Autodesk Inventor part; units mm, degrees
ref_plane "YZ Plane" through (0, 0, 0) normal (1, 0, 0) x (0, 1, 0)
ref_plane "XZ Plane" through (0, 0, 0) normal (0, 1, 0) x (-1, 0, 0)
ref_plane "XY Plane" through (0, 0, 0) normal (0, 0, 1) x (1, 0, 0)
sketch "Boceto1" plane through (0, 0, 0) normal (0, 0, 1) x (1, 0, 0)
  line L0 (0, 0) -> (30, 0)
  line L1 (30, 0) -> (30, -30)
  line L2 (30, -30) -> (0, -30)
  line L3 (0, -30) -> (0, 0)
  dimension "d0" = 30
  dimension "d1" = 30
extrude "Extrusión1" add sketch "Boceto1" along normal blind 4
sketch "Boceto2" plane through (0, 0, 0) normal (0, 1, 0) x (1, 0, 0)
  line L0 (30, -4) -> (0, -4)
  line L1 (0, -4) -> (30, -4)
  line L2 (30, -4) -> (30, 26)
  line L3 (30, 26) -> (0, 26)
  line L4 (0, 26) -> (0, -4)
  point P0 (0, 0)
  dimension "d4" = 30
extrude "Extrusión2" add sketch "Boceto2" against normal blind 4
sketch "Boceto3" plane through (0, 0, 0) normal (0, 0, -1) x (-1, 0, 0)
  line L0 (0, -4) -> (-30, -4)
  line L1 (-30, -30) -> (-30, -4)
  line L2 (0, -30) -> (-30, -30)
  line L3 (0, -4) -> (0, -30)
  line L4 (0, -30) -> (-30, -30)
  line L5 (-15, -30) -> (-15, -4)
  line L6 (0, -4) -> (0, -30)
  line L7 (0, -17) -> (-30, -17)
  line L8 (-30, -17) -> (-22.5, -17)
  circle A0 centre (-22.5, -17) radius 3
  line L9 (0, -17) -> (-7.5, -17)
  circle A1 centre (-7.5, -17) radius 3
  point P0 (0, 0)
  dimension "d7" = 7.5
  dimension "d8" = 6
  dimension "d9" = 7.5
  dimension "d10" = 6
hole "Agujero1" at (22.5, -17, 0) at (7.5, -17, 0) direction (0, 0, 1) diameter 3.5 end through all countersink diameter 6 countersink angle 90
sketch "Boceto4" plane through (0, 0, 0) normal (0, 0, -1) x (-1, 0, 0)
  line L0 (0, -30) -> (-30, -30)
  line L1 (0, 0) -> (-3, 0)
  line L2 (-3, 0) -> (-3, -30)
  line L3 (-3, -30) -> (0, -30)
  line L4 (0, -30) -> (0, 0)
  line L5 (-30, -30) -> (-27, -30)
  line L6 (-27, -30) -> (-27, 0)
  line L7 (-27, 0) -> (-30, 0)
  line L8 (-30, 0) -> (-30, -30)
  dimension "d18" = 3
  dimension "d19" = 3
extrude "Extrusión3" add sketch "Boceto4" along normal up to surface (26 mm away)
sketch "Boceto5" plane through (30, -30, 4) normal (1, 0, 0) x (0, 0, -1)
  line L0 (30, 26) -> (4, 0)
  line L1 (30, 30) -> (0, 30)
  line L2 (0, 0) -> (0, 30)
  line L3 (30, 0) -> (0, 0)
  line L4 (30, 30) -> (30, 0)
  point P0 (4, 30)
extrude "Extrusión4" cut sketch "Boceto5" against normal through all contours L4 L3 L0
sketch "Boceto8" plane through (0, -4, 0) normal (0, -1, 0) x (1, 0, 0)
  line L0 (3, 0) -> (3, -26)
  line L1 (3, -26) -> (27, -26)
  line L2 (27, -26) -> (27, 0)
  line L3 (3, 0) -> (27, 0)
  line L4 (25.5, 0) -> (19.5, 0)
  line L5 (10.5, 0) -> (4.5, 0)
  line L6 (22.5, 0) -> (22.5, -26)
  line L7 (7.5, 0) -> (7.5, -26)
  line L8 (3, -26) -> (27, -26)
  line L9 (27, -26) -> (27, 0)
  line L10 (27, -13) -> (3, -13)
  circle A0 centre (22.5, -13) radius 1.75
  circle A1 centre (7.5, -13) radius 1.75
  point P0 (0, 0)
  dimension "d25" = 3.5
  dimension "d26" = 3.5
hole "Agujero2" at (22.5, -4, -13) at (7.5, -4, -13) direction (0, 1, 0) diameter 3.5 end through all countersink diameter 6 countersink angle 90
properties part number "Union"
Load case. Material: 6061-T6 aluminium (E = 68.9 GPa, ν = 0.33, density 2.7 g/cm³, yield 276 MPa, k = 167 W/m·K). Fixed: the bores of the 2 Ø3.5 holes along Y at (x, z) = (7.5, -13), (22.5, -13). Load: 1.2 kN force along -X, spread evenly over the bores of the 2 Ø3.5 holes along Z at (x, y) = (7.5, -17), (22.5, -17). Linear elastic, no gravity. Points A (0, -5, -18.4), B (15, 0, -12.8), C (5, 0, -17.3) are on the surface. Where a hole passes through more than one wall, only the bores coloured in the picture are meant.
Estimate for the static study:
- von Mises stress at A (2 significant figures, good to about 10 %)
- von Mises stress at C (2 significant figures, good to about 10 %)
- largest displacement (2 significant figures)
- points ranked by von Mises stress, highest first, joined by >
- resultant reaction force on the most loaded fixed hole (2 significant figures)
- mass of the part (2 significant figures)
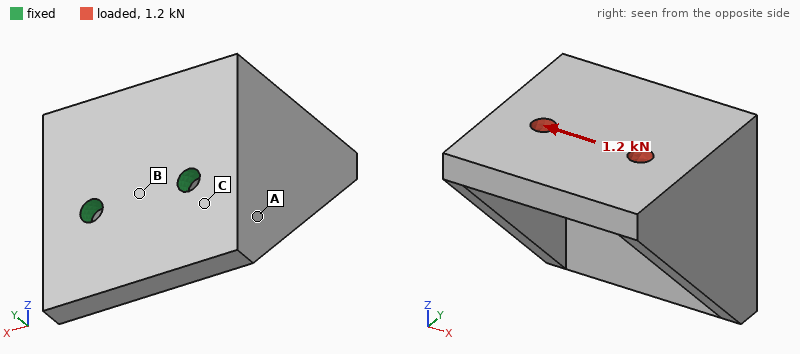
41 MPa
63 MPa
0.15 mm
C > A > B
1.5 kN
23 g
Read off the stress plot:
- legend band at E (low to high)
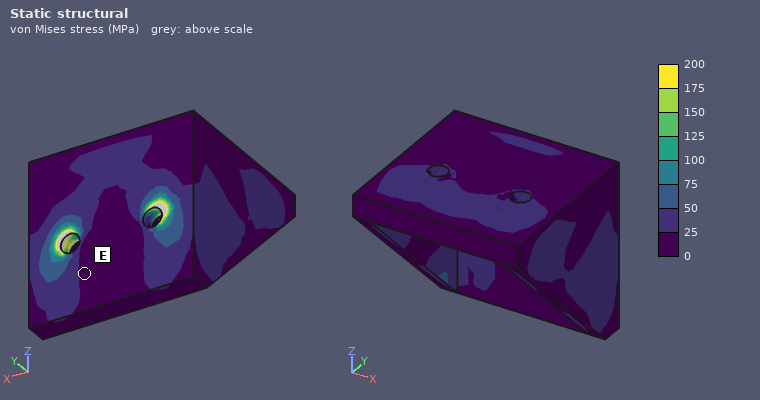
0 to 25 MPa
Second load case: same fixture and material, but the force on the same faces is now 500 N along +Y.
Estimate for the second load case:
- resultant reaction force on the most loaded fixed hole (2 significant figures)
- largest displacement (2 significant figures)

250 N
89 µm
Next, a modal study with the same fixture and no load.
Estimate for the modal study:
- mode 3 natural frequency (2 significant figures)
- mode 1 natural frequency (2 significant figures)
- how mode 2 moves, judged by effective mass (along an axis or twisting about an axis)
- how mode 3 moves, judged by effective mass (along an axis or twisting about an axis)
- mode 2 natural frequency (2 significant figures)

12 kHz
3400 Hz
along X
along X
4600 Hz
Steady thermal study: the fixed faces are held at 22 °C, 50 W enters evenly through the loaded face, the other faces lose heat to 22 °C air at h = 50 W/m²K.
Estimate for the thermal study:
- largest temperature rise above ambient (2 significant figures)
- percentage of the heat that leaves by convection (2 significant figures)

50 K
12 %
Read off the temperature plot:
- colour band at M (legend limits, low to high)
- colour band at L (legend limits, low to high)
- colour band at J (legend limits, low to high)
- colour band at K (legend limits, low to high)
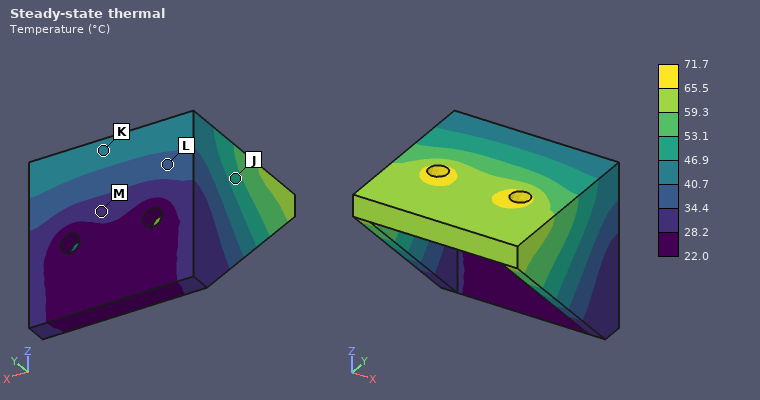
28.2 to 34.4 °C
34.4 to 40.7 °C
46.9 to 53.1 °C
40.7 to 46.9 °C
